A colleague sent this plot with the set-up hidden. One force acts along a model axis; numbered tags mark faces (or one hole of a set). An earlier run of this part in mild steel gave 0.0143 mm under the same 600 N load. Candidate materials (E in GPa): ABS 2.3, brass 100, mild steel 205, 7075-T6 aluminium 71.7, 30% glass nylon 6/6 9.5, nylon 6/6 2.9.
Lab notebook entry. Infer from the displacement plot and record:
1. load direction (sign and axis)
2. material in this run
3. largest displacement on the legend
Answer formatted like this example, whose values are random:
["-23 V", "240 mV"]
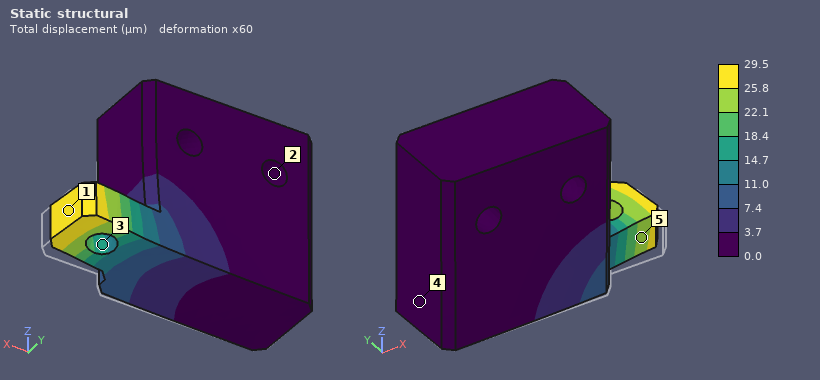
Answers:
["+Y", "brass", "29.5 µm"]
